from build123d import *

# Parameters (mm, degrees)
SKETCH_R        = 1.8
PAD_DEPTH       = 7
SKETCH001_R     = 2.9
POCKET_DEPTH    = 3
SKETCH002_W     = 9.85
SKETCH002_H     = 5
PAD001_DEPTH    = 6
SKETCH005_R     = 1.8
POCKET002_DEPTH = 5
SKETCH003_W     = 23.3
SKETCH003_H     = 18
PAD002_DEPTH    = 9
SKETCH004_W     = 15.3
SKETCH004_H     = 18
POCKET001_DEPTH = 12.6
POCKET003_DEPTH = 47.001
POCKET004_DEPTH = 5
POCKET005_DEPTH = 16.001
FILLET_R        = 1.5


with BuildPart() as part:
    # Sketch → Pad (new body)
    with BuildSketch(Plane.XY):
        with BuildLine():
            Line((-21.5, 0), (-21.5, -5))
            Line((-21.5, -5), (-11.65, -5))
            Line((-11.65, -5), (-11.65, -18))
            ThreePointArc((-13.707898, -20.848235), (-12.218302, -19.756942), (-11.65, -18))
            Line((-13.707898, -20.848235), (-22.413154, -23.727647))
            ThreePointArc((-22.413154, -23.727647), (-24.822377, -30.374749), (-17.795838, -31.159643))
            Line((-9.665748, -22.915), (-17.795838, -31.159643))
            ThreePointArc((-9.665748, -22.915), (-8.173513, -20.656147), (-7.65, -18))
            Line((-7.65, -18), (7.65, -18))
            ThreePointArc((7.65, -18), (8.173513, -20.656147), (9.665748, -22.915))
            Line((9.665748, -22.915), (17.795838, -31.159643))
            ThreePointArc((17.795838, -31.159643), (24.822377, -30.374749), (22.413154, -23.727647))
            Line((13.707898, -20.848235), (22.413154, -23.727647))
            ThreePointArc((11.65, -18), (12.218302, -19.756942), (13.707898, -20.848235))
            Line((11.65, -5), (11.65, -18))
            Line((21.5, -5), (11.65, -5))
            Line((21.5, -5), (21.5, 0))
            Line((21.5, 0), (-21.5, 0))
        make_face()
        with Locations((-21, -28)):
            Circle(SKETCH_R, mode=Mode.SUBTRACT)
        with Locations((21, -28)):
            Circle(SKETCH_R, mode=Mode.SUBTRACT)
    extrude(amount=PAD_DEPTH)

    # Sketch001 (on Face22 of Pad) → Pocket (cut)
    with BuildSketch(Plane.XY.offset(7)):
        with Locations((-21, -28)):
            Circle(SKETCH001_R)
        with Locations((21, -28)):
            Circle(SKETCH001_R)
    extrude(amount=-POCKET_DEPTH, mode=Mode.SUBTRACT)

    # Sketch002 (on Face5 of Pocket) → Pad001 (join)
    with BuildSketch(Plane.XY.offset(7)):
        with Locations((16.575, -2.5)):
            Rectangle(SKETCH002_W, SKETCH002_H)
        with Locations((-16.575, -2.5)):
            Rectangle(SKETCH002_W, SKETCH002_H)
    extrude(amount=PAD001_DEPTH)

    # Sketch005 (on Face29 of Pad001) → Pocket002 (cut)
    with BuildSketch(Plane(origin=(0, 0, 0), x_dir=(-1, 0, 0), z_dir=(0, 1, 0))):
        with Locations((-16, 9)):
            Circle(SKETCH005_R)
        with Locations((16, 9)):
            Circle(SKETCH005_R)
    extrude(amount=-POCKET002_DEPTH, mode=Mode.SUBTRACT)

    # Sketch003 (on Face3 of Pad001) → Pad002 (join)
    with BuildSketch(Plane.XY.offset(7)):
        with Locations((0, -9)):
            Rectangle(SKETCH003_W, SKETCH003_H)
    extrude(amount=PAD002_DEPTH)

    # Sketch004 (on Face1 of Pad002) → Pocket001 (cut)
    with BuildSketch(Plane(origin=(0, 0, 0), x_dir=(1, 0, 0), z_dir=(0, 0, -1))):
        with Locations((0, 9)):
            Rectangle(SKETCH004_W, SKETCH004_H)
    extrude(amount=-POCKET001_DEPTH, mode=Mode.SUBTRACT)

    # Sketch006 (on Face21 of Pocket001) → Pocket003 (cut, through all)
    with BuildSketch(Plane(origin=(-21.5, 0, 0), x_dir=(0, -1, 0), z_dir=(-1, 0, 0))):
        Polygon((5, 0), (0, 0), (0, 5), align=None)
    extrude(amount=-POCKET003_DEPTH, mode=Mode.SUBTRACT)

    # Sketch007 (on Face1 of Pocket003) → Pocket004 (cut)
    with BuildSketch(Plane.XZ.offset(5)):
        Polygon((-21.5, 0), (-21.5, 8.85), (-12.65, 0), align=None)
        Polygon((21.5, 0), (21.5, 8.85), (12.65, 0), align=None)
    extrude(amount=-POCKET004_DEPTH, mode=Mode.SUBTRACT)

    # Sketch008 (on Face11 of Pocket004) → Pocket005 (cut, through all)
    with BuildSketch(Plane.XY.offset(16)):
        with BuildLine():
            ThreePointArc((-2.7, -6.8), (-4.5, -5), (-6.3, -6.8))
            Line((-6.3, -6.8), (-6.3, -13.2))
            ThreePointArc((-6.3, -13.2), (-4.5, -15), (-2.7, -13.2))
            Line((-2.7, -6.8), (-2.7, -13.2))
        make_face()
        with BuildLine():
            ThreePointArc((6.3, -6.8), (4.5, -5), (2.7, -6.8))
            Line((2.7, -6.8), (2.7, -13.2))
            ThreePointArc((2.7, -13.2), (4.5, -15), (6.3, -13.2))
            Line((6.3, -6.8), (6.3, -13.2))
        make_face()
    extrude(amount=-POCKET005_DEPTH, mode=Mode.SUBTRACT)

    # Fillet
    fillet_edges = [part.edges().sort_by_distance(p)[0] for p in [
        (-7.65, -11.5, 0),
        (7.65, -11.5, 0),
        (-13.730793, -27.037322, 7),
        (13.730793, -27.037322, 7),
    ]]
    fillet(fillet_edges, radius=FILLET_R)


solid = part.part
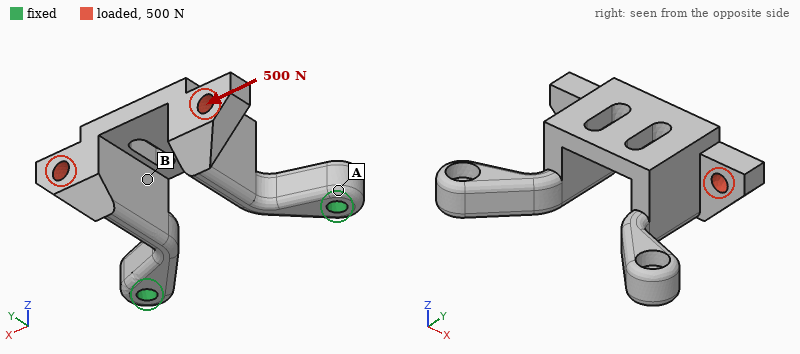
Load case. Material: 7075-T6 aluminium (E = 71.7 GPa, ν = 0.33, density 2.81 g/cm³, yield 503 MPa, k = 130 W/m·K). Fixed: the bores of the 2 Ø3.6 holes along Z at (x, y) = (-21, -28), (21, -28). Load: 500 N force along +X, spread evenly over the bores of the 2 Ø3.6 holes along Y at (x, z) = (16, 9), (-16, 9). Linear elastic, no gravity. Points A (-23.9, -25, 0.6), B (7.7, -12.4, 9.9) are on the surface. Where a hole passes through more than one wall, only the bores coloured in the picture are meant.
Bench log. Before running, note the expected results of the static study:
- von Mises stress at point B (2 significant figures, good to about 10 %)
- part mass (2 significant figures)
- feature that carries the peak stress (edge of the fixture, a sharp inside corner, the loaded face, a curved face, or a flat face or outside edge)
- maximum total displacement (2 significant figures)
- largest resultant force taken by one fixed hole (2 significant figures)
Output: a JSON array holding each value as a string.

["45 MPa", "14 g", "a curved face", "0.13 mm", "410 N"]
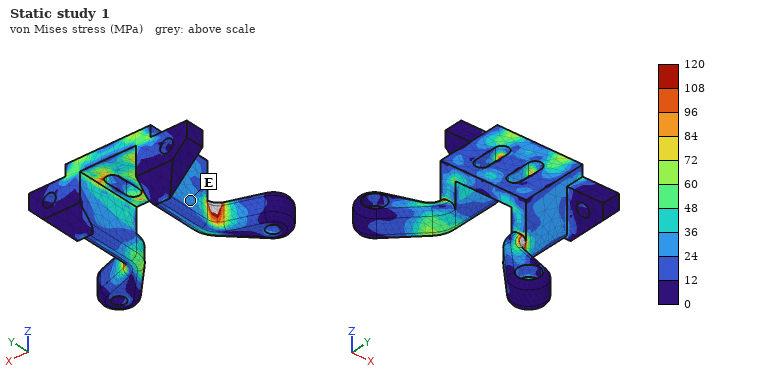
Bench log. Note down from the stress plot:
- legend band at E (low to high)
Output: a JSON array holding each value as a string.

["24 to 36 MPa"]
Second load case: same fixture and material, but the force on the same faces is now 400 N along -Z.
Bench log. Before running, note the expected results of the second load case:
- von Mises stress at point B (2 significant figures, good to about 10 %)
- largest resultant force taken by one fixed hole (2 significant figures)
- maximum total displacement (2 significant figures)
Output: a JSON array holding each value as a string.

["26 MPa", "210 N", "0.35 mm"]
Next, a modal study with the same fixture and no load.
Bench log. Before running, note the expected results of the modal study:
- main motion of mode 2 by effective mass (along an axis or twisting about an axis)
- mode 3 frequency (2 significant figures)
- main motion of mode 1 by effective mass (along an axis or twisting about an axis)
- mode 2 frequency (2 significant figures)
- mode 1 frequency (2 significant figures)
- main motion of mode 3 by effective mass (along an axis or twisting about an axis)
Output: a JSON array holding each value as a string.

["along X", "6000 Hz", "along Z", "3900 Hz", "2200 Hz", "along X"]
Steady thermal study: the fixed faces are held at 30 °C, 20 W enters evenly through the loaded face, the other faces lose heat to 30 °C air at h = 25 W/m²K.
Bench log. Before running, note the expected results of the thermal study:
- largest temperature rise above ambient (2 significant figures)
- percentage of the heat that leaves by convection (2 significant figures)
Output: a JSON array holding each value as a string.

["63 K", "16 %"]
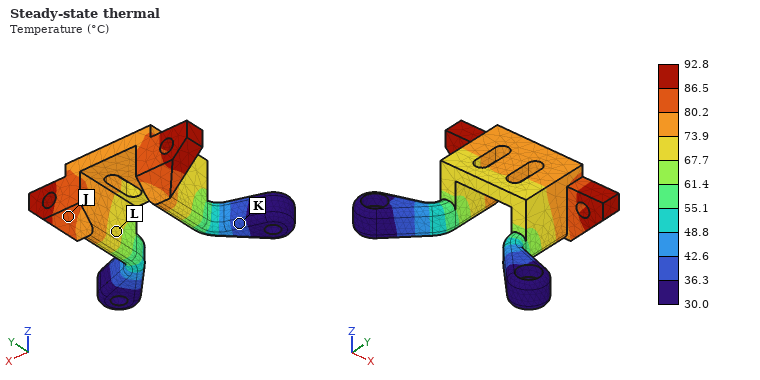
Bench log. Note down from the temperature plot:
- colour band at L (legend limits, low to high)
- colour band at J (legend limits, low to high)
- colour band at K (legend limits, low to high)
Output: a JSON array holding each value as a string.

["67.7 to 73.9 °C", "80.2 to 86.5 °C", "36.3 to 42.6 °C"]
